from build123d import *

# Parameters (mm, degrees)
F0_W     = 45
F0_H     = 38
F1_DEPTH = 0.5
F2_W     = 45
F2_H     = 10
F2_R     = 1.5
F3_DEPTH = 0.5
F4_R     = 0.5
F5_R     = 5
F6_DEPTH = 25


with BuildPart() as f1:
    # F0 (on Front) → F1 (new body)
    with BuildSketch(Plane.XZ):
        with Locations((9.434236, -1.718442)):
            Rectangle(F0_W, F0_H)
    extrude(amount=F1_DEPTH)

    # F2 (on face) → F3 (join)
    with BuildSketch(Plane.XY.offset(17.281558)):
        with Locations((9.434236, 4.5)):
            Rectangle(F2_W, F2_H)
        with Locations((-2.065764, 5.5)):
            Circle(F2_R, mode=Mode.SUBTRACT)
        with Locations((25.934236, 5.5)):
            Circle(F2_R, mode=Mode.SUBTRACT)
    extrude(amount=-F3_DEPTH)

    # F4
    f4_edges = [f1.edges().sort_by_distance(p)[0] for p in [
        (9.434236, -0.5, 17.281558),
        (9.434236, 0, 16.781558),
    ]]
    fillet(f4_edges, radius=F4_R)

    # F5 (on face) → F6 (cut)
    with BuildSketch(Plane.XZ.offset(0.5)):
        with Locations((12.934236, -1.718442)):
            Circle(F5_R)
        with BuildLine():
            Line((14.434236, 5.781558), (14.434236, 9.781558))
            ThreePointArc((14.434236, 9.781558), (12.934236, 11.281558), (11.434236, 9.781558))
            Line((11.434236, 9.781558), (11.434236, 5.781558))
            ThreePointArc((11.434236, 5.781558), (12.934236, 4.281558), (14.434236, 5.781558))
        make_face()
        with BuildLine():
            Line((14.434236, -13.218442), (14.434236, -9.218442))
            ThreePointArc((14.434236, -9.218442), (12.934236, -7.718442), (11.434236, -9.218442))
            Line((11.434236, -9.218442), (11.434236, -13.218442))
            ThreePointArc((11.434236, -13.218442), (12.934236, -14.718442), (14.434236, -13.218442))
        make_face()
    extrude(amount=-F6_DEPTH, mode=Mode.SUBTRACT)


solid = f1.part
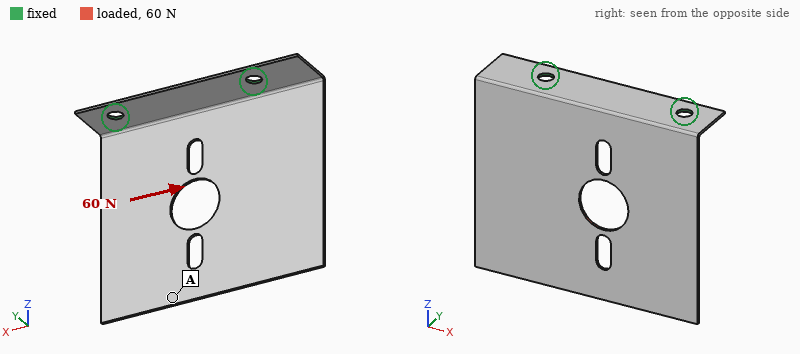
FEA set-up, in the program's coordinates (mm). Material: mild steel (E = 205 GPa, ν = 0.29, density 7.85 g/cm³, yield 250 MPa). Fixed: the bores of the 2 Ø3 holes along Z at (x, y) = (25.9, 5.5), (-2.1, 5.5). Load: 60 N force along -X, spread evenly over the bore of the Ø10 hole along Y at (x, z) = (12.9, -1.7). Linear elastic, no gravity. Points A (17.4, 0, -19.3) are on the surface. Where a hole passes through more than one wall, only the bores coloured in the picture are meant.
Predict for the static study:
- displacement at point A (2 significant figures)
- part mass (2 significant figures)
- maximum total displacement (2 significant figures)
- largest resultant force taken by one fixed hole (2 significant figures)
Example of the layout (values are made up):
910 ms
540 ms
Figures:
0.11 mm
7.9 g
0.23 mm
50 N
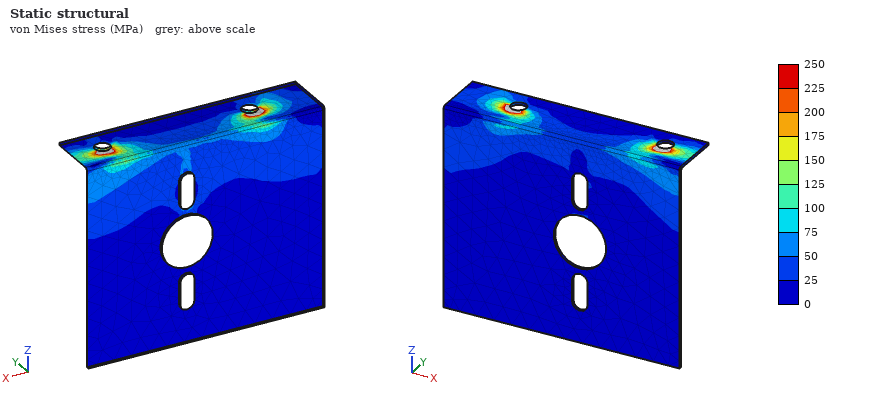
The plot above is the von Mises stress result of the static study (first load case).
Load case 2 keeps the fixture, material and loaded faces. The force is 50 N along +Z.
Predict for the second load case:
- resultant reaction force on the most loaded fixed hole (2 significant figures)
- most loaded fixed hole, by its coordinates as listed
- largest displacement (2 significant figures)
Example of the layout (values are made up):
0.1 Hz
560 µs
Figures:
27 N
(25.9, 5.5)
0.34 mm
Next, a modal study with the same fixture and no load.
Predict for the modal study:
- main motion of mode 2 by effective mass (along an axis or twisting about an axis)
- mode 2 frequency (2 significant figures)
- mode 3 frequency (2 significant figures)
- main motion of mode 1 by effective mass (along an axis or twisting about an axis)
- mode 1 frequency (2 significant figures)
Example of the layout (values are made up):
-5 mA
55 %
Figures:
twisting about Z
550 Hz
1400 Hz
along Y
230 Hz
